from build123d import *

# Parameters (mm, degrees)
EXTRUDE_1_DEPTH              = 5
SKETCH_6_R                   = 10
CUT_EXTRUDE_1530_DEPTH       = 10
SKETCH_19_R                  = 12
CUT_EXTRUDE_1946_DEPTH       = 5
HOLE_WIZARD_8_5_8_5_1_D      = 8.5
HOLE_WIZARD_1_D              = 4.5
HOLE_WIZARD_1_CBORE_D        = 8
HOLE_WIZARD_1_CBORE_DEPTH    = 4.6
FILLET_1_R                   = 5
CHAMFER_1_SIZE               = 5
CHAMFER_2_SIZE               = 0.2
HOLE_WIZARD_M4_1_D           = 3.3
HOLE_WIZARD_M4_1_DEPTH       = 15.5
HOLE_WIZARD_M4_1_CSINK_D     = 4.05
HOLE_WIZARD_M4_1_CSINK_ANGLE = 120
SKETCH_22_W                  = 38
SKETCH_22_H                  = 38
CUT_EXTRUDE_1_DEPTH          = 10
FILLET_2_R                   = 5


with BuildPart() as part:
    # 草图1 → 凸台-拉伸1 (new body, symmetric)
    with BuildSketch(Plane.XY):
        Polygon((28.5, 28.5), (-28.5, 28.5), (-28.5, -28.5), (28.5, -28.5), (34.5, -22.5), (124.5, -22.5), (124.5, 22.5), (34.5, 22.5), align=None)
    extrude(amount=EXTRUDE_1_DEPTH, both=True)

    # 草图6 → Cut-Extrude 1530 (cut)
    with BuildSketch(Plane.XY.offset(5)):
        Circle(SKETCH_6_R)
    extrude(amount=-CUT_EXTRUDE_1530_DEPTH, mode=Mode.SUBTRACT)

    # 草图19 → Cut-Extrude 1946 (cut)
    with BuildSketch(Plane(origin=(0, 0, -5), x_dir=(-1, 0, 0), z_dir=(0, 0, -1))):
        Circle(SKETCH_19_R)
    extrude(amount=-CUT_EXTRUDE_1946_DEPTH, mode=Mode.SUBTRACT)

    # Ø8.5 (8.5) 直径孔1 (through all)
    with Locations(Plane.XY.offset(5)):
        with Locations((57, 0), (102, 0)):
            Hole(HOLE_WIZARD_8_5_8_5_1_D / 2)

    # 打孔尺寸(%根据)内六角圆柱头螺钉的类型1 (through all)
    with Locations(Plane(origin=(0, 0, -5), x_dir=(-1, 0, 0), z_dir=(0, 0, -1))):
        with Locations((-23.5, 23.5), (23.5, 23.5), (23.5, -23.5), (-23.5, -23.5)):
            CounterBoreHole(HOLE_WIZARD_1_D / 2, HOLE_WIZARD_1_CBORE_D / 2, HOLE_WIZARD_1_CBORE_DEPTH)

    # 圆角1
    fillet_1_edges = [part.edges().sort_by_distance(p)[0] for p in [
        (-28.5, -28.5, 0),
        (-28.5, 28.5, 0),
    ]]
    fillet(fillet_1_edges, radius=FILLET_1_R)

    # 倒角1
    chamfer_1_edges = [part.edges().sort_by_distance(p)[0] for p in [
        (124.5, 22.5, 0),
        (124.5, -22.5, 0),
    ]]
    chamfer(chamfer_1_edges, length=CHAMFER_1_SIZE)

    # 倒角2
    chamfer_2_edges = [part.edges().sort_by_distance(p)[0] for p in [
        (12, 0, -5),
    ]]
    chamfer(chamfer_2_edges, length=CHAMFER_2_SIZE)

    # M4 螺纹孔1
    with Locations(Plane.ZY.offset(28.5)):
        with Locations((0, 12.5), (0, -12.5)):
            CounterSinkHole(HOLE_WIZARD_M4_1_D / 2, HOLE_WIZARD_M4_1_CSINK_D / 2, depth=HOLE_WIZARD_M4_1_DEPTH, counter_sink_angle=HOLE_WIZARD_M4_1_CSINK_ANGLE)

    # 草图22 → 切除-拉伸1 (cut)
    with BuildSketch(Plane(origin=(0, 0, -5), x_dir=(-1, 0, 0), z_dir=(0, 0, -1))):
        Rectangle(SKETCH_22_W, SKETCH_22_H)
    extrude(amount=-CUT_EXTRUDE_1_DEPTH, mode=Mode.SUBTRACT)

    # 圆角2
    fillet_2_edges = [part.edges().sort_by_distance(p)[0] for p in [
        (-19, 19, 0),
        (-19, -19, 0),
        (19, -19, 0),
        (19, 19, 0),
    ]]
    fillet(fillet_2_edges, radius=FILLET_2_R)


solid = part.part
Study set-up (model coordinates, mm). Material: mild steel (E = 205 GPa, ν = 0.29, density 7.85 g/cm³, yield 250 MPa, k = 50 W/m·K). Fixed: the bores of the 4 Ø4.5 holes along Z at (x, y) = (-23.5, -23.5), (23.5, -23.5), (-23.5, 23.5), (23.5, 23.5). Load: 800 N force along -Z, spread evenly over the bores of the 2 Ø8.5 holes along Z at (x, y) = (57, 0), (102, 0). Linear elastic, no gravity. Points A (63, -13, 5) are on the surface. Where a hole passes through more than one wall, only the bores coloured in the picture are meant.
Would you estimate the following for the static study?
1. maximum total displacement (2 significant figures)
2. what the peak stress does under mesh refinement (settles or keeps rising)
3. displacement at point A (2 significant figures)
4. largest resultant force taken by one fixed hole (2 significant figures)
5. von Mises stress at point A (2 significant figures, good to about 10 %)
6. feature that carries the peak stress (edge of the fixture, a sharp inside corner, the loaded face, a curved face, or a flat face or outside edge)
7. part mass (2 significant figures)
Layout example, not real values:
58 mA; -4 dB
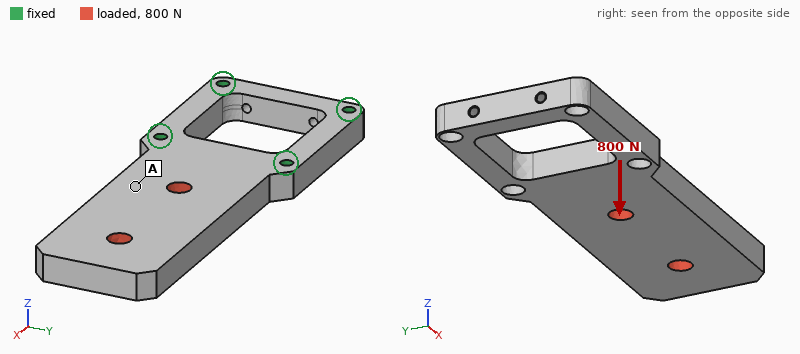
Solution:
0.26 mm; keeps rising; 0.078 mm; 790 N; 24 MPa; edge of the fixture; 460 g
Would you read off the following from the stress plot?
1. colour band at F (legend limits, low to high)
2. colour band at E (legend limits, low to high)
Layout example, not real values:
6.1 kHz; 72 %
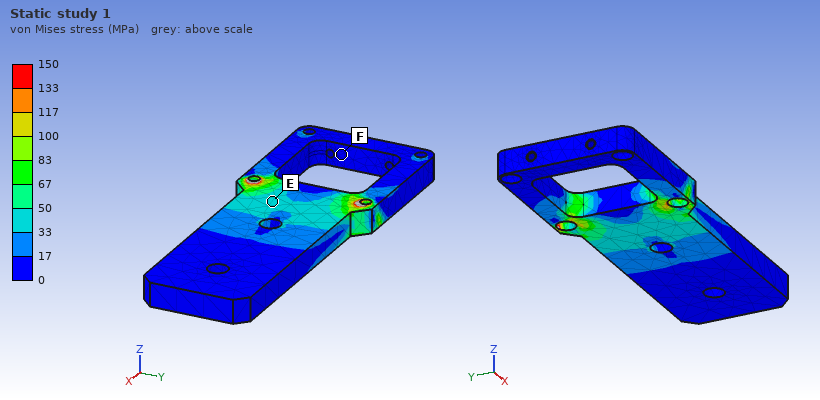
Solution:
0 to 17 MPa; 33 to 50 MPa
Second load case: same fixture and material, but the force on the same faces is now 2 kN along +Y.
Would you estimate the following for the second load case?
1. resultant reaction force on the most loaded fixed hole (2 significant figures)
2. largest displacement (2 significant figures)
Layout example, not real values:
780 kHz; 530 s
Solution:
2.5 kN; 25 µm
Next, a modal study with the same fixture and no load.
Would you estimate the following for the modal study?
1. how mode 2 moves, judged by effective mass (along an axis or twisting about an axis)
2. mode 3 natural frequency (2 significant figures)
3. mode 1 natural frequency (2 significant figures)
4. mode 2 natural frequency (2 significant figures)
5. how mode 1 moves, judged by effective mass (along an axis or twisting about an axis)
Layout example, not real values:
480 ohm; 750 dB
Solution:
along Y; 3400 Hz; 620 Hz; 3100 Hz; along Z
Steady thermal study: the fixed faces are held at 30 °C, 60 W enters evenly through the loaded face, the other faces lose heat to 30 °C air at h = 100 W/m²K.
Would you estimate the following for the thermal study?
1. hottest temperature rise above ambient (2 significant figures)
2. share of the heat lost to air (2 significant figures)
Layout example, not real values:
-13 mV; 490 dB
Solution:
60 K; 72 %
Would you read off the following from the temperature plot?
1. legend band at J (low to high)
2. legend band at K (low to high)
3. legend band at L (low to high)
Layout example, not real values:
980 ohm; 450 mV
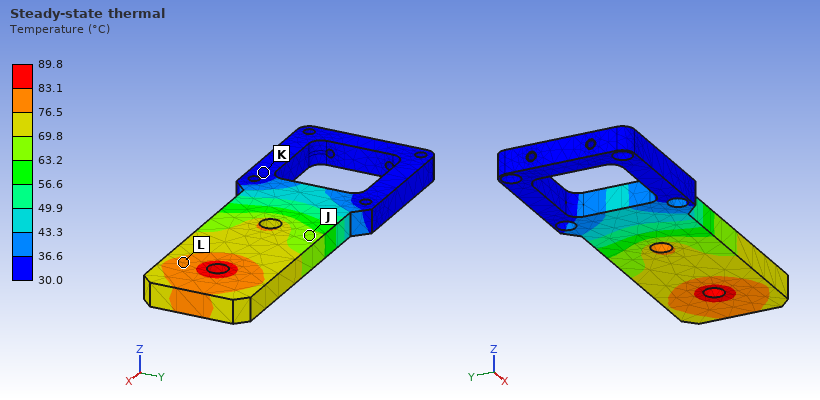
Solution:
63.2 to 69.8 °C; 30.0 to 36.6 °C; 76.5 to 83.1 °C
